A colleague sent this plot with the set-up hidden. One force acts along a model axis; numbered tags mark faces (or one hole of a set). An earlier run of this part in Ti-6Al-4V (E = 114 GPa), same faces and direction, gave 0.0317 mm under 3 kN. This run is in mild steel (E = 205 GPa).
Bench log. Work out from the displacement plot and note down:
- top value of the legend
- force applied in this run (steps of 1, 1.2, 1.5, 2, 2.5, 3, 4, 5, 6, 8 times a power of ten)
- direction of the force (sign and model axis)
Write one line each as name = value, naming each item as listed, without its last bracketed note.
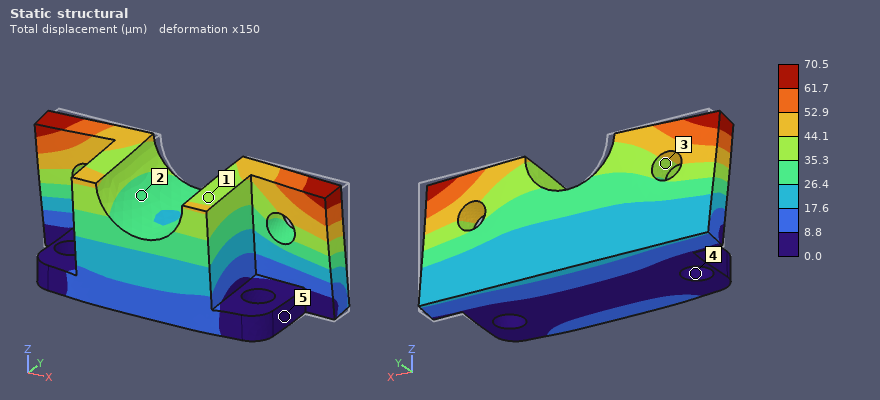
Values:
top value of the legend = 70.5 µm
force applied in this run = 12 kN
direction of the force = -Y
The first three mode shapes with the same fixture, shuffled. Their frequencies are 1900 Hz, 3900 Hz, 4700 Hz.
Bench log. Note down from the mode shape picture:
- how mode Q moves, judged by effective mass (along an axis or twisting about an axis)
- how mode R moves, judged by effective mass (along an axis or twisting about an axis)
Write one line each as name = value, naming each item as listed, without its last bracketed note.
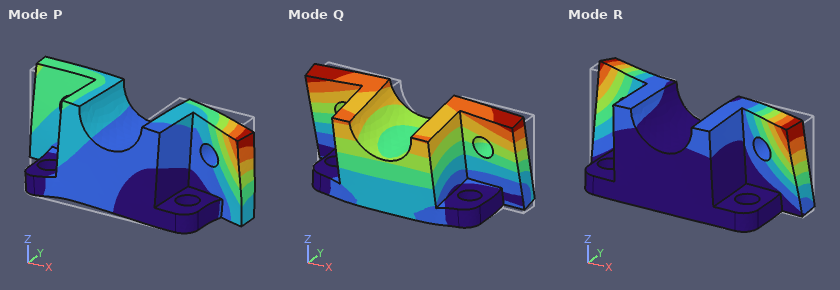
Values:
how mode Q moves, judged by effective mass = along Y
how mode R moves, judged by effective mass = twisting about Z
